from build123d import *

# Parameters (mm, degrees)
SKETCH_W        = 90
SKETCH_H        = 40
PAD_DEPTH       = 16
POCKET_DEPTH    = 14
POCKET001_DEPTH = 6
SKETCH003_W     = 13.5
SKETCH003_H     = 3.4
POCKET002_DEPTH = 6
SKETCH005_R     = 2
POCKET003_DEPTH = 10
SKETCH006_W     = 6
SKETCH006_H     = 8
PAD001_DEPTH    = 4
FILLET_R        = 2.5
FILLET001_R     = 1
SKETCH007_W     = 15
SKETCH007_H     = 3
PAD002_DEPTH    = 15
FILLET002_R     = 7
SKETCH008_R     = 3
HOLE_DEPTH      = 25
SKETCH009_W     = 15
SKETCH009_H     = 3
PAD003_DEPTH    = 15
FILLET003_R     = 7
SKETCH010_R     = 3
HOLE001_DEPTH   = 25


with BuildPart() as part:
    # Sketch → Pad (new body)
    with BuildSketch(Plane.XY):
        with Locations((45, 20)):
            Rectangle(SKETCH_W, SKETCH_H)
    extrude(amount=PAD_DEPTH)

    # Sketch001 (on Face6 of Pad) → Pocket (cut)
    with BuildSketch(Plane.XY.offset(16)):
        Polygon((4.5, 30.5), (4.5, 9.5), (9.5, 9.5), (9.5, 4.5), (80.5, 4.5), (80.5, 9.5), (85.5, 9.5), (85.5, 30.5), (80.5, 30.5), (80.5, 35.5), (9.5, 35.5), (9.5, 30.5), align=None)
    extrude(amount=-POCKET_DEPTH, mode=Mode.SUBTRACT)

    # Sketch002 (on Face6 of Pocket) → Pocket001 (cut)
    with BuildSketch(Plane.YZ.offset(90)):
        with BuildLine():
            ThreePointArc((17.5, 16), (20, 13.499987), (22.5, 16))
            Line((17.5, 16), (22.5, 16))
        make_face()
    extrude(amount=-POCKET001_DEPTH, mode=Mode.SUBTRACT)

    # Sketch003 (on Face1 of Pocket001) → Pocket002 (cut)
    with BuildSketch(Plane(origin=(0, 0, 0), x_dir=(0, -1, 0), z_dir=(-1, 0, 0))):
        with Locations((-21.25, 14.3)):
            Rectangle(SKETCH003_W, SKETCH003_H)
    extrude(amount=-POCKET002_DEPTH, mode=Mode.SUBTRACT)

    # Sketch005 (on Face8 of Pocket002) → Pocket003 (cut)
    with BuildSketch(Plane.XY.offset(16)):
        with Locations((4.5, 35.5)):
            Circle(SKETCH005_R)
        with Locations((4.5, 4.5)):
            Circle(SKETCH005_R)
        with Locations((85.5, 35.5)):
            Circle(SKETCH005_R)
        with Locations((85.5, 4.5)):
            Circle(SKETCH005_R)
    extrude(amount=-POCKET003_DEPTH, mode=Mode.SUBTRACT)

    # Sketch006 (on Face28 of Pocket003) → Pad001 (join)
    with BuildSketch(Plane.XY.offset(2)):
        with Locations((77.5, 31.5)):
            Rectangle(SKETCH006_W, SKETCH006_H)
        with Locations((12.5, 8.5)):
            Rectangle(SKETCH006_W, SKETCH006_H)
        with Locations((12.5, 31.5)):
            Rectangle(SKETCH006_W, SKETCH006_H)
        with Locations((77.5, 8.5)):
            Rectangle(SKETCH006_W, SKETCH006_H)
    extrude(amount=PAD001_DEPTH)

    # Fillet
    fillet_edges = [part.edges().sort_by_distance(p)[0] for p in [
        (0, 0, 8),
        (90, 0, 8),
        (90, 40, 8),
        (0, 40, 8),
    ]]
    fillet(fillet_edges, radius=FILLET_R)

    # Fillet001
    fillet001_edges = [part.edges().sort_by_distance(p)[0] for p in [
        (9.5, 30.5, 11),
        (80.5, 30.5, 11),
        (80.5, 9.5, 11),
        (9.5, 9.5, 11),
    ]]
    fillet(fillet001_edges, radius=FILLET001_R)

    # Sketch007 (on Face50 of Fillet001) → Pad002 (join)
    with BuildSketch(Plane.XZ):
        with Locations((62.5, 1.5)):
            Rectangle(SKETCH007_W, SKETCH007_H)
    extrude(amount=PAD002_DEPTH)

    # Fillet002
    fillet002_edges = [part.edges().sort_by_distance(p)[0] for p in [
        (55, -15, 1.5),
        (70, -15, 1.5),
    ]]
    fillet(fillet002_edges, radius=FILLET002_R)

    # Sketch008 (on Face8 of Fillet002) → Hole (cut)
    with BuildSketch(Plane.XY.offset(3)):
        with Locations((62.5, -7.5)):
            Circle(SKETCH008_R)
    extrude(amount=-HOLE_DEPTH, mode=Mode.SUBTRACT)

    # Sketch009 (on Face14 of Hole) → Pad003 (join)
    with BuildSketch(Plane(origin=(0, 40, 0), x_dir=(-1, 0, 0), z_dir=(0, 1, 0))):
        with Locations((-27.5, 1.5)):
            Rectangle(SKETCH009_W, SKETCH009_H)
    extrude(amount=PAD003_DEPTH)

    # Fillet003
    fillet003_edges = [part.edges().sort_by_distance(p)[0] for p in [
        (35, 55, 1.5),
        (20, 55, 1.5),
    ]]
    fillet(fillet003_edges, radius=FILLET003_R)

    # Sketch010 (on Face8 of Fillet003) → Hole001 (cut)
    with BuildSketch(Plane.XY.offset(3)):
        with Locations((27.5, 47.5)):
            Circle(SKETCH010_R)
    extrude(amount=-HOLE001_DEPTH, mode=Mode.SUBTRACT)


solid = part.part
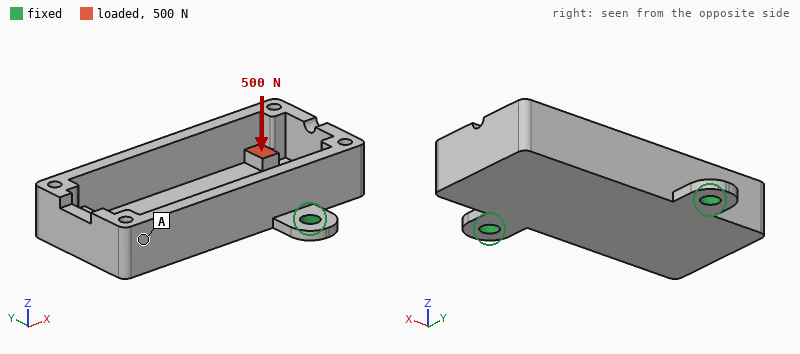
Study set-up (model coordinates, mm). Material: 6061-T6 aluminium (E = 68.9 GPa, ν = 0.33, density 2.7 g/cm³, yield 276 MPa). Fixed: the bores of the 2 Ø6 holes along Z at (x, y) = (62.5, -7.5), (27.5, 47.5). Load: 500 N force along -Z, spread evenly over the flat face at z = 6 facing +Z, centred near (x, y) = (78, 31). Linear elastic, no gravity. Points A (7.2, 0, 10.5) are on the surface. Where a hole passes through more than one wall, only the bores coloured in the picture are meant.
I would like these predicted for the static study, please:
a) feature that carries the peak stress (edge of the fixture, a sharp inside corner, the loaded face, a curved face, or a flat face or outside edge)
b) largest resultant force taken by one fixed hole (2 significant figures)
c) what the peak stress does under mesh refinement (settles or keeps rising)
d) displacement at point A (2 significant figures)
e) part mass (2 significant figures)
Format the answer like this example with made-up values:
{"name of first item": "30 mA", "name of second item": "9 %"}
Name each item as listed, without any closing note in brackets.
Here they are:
{"feature that carries the peak stress": "edge of the fixture", "largest resultant force taken by one fixed hole": "290 N", "what the peak stress does under mesh refinement": "keeps rising", "displacement at point A": "0.49 mm", "part mass": "67 g"}
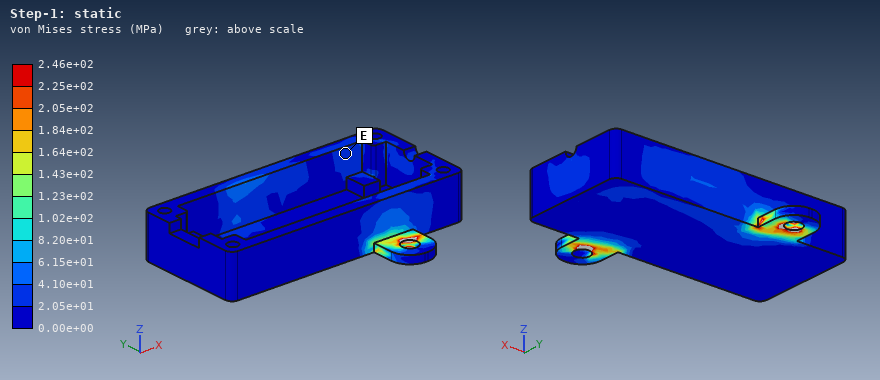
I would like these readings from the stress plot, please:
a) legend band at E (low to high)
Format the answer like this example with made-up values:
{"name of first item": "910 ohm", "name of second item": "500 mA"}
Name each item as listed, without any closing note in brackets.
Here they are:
{"legend band at E": "2.05e+01 to 4.10e+01 MPa"}
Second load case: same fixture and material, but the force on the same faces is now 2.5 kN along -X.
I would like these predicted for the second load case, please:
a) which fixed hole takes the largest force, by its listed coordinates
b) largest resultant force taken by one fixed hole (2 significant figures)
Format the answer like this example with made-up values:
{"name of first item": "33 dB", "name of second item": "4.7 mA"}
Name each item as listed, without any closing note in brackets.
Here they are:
{"which fixed hole takes the largest force, by its listed coordinates": "(27.5, 47.5)", "largest resultant force taken by one fixed hole": "1.7 kN"}
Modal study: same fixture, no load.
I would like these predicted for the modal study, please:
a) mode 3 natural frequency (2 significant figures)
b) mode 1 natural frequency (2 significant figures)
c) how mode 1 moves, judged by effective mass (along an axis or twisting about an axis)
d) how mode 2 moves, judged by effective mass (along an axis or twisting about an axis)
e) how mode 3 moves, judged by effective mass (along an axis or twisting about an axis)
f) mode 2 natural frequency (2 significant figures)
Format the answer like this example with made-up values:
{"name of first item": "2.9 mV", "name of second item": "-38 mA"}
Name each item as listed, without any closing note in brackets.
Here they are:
{"mode 3 natural frequency": "5000 Hz", "mode 1 natural frequency": "840 Hz", "how mode 1 moves, judged by effective mass": "twisting about Y", "how mode 2 moves, judged by effective mass": "along Z", "how mode 3 moves, judged by effective mass": "along Z", "mode 2 natural frequency": "2100 Hz"}
